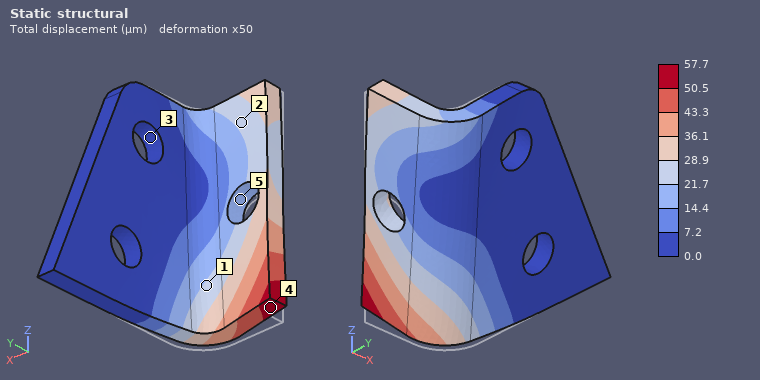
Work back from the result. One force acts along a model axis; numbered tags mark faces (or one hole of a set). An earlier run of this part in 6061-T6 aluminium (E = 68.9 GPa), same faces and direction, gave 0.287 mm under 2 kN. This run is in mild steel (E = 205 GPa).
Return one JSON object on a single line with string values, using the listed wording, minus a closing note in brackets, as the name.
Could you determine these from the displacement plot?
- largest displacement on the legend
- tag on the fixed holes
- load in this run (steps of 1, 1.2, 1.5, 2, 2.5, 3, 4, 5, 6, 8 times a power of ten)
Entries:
{"largest displacement on the legend": "57.7 µm", "tag on the fixed holes": "3", "load in this run": "1.2 kN"}
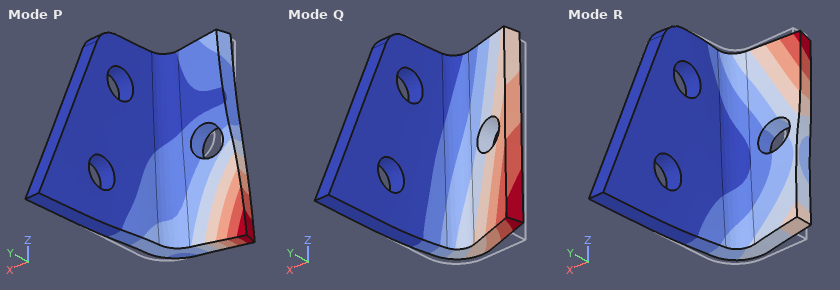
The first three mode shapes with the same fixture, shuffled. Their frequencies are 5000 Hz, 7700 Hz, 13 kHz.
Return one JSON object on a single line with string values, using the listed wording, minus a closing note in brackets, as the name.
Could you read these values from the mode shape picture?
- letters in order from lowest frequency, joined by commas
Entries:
{"letters in order from lowest frequency, joined by commas": "Q, R, P"}
